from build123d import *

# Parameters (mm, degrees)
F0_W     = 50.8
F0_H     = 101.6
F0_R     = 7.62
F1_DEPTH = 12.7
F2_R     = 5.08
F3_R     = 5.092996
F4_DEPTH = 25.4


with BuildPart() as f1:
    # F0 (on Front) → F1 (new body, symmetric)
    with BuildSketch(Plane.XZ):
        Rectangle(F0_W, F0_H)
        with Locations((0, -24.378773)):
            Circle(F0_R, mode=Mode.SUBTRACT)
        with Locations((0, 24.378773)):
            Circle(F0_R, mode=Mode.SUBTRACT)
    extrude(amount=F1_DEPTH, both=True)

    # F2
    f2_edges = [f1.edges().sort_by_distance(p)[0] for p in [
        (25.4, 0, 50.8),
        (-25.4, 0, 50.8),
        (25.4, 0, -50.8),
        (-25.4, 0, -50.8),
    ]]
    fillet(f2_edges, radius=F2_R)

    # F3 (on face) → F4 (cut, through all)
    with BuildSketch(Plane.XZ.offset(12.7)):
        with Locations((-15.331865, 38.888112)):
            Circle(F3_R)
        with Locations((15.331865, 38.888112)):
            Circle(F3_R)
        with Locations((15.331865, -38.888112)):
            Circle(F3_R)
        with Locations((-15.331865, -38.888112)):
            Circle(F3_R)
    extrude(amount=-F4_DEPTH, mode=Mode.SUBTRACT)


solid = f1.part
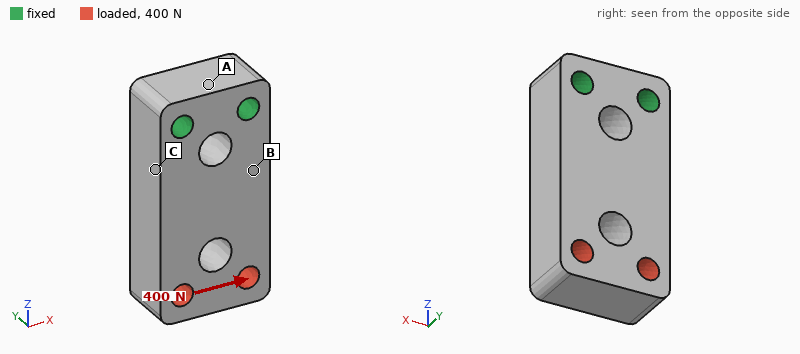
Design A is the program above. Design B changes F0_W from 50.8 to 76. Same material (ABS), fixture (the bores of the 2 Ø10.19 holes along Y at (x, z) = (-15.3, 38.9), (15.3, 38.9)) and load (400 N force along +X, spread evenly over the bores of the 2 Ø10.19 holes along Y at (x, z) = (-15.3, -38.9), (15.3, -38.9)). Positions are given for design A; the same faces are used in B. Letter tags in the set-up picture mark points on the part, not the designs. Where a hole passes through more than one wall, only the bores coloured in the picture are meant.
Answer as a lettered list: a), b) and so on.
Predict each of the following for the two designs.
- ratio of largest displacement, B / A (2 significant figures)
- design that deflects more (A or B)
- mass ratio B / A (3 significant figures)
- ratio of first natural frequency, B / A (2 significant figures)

a) 0.66
b) A
c) 1.58
d) 0.94
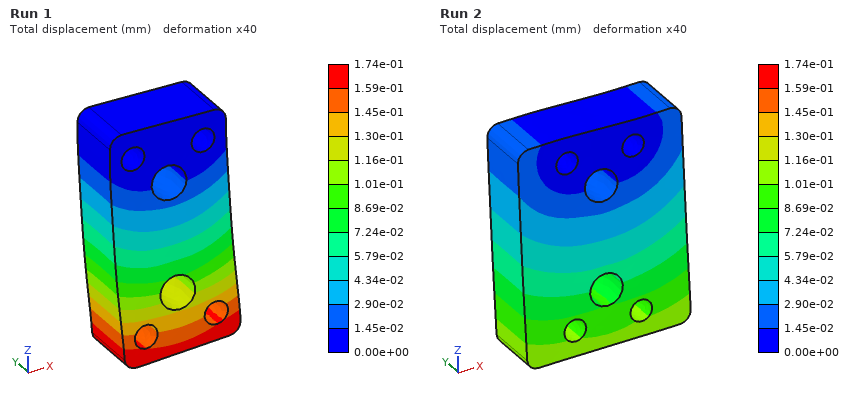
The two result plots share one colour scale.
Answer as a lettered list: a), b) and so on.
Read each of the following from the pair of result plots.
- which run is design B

a) Run 2
